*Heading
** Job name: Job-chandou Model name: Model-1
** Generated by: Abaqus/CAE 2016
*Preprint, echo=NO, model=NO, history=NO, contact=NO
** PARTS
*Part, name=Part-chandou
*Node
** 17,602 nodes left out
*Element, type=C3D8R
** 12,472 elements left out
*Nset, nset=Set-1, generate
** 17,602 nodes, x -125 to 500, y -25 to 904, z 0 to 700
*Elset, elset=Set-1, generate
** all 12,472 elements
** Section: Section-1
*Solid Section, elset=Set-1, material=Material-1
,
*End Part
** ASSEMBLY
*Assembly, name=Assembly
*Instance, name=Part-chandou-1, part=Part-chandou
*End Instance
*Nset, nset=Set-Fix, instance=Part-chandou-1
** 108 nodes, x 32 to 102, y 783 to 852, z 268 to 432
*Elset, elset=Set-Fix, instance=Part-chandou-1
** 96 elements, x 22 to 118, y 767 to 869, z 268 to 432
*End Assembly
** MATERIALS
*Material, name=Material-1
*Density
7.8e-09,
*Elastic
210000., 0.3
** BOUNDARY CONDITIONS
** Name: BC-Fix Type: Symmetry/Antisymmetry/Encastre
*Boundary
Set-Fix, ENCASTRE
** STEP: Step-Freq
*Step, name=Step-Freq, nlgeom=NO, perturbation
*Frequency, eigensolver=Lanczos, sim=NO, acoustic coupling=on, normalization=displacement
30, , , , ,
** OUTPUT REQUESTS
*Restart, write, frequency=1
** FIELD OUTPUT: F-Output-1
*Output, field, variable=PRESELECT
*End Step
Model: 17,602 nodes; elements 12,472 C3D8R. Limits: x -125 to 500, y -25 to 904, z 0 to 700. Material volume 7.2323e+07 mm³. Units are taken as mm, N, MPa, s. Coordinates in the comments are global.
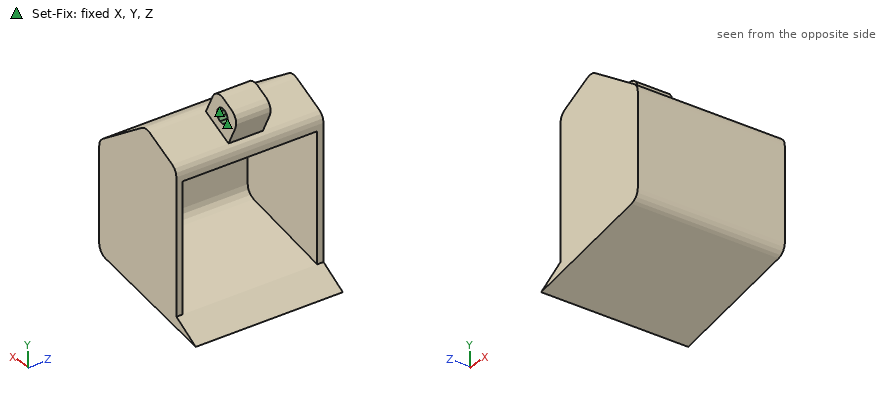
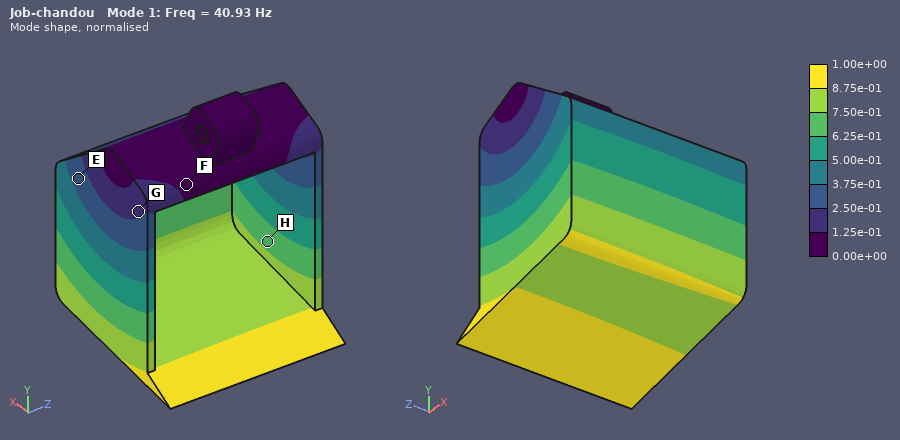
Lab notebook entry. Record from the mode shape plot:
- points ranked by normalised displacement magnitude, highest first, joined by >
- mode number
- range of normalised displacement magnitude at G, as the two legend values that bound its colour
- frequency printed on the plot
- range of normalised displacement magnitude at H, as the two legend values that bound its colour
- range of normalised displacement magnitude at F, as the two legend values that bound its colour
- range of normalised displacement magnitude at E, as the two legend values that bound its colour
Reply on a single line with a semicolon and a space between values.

H > E > G > F; 1; 1.25e-01 to 2.50e-01; 40.93 Hz; 6.25e-01 to 7.50e-01; 0.00e+00 to 1.25e-01; 2.50e-01 to 3.75e-01
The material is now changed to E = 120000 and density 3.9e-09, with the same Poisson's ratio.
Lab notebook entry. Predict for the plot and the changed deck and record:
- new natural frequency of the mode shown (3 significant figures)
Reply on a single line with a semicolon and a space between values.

43.8 Hz
